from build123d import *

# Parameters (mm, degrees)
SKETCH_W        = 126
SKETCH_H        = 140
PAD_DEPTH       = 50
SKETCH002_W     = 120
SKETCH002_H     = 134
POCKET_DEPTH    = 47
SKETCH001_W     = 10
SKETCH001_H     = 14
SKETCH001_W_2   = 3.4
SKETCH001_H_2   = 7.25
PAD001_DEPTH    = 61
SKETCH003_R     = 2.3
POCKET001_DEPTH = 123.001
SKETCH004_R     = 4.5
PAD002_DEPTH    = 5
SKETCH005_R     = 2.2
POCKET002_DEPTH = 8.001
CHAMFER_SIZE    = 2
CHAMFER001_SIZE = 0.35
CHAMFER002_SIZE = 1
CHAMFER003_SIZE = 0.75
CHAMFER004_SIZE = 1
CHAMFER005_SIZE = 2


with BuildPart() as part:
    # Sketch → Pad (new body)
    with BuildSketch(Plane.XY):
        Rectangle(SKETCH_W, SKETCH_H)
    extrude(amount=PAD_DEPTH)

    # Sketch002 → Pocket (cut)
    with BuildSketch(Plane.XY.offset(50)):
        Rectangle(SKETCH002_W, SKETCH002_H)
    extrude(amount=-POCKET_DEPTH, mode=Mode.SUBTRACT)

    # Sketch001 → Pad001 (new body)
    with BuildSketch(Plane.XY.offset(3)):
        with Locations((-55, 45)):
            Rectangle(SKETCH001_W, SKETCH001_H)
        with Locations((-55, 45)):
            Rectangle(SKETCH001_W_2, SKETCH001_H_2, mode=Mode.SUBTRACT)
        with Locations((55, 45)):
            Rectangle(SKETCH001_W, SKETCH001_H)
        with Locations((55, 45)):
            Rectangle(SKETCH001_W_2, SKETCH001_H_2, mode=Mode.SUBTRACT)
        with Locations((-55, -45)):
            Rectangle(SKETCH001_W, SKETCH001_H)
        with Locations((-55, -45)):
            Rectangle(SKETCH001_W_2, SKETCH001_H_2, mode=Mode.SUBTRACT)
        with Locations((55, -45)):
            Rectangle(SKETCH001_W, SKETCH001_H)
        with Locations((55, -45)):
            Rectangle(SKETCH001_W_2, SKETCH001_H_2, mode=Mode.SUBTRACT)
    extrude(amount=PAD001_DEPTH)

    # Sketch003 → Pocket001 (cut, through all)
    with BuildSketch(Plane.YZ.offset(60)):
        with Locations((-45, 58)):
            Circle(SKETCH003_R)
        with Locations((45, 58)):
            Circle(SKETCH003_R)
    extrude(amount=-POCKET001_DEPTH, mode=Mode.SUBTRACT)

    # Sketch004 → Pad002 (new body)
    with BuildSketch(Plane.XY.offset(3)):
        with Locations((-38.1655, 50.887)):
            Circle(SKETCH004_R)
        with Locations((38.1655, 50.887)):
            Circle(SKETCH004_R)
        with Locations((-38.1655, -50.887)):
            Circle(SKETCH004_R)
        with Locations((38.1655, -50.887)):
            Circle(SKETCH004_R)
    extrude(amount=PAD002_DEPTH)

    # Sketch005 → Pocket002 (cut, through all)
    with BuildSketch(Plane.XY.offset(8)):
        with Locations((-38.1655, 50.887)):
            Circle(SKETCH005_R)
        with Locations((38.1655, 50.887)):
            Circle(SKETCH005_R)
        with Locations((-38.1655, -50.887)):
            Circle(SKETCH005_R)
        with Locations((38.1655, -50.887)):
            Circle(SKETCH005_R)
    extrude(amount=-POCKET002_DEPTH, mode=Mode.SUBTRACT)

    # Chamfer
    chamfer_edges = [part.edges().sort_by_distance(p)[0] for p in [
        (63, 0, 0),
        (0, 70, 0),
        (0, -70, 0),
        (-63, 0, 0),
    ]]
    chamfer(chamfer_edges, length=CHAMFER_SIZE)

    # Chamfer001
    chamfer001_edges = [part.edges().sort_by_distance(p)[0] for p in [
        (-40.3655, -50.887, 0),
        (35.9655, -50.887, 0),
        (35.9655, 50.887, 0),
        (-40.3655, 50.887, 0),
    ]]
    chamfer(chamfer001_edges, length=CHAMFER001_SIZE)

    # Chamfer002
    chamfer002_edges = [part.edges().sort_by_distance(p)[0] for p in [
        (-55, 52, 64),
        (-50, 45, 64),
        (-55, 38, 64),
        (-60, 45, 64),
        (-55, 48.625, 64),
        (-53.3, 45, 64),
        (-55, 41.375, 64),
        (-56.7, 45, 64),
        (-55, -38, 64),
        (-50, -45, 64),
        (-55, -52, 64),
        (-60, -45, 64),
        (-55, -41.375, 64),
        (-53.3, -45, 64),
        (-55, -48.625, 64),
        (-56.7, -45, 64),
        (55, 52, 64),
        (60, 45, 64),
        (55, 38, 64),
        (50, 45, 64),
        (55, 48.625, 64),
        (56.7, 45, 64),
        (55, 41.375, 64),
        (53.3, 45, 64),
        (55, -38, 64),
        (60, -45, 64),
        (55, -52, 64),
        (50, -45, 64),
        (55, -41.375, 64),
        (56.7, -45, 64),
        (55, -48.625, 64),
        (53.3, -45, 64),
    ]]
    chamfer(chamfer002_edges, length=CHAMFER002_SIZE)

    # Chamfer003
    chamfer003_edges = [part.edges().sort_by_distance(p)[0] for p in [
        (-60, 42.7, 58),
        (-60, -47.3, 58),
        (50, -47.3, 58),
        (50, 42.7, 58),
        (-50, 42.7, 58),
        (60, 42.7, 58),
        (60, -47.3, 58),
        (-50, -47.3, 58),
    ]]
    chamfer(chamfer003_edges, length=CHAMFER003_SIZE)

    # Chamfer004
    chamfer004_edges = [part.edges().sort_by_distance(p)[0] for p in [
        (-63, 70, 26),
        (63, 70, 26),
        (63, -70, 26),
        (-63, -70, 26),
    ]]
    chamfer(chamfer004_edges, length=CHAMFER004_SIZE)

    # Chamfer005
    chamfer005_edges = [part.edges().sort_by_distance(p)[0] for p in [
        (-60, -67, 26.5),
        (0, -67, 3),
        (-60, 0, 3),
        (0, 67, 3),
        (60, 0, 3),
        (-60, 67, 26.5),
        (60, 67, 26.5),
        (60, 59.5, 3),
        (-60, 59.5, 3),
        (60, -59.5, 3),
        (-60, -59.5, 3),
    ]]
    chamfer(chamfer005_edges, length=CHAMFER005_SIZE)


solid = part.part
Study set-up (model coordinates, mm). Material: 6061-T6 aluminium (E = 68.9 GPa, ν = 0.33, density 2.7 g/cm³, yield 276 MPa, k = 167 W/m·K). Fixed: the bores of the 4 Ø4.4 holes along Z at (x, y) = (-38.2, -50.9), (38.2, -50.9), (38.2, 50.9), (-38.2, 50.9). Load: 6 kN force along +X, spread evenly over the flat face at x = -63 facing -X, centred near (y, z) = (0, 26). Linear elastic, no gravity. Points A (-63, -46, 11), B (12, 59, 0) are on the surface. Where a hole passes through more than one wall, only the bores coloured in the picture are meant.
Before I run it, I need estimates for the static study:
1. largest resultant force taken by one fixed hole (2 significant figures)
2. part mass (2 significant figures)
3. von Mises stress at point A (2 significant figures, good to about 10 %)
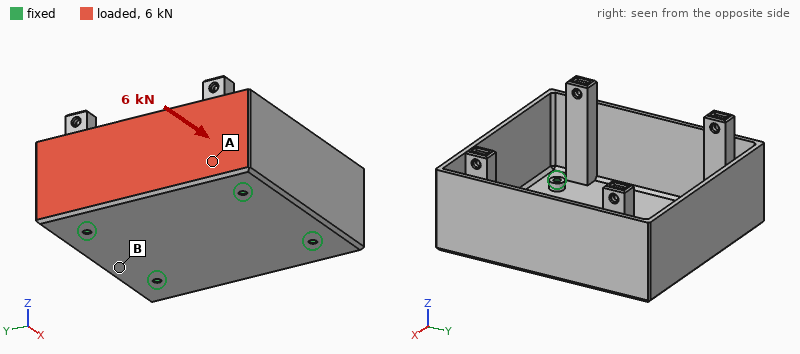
1.9 kN
420 g
100 MPa
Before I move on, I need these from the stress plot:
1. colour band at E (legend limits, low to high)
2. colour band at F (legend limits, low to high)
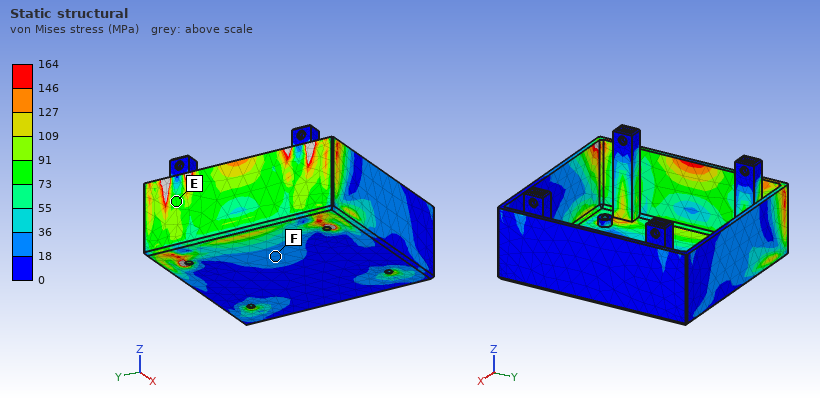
73 to 91 MPa
18 to 36 MPa
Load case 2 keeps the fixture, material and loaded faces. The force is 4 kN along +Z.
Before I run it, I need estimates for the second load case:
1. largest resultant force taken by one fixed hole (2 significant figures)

2.5 kN
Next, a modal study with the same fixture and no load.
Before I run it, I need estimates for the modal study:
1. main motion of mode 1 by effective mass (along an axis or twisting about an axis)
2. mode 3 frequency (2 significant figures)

along X
1500 Hz
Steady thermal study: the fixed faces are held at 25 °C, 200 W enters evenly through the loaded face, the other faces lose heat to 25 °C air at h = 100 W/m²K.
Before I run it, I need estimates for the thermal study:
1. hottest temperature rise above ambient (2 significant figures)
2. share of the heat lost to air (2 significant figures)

72 K
64 %
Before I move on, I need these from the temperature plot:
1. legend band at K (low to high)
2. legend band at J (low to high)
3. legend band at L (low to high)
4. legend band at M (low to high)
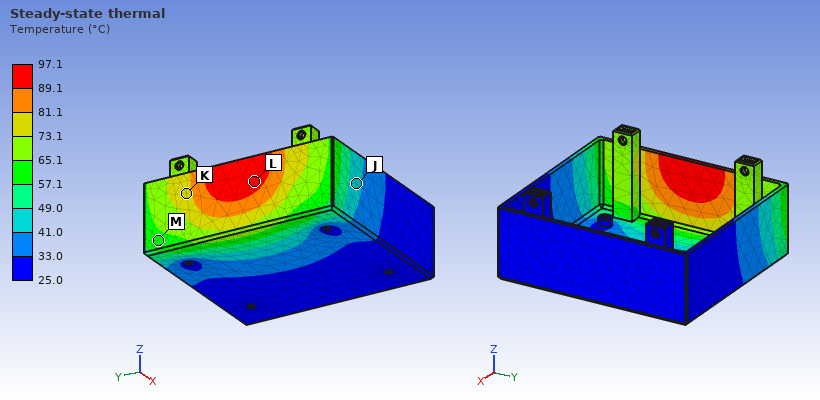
73.1 to 81.1 °C
41.0 to 49.0 °C
89.1 to 97.1 °C
57.1 to 65.1 °C
